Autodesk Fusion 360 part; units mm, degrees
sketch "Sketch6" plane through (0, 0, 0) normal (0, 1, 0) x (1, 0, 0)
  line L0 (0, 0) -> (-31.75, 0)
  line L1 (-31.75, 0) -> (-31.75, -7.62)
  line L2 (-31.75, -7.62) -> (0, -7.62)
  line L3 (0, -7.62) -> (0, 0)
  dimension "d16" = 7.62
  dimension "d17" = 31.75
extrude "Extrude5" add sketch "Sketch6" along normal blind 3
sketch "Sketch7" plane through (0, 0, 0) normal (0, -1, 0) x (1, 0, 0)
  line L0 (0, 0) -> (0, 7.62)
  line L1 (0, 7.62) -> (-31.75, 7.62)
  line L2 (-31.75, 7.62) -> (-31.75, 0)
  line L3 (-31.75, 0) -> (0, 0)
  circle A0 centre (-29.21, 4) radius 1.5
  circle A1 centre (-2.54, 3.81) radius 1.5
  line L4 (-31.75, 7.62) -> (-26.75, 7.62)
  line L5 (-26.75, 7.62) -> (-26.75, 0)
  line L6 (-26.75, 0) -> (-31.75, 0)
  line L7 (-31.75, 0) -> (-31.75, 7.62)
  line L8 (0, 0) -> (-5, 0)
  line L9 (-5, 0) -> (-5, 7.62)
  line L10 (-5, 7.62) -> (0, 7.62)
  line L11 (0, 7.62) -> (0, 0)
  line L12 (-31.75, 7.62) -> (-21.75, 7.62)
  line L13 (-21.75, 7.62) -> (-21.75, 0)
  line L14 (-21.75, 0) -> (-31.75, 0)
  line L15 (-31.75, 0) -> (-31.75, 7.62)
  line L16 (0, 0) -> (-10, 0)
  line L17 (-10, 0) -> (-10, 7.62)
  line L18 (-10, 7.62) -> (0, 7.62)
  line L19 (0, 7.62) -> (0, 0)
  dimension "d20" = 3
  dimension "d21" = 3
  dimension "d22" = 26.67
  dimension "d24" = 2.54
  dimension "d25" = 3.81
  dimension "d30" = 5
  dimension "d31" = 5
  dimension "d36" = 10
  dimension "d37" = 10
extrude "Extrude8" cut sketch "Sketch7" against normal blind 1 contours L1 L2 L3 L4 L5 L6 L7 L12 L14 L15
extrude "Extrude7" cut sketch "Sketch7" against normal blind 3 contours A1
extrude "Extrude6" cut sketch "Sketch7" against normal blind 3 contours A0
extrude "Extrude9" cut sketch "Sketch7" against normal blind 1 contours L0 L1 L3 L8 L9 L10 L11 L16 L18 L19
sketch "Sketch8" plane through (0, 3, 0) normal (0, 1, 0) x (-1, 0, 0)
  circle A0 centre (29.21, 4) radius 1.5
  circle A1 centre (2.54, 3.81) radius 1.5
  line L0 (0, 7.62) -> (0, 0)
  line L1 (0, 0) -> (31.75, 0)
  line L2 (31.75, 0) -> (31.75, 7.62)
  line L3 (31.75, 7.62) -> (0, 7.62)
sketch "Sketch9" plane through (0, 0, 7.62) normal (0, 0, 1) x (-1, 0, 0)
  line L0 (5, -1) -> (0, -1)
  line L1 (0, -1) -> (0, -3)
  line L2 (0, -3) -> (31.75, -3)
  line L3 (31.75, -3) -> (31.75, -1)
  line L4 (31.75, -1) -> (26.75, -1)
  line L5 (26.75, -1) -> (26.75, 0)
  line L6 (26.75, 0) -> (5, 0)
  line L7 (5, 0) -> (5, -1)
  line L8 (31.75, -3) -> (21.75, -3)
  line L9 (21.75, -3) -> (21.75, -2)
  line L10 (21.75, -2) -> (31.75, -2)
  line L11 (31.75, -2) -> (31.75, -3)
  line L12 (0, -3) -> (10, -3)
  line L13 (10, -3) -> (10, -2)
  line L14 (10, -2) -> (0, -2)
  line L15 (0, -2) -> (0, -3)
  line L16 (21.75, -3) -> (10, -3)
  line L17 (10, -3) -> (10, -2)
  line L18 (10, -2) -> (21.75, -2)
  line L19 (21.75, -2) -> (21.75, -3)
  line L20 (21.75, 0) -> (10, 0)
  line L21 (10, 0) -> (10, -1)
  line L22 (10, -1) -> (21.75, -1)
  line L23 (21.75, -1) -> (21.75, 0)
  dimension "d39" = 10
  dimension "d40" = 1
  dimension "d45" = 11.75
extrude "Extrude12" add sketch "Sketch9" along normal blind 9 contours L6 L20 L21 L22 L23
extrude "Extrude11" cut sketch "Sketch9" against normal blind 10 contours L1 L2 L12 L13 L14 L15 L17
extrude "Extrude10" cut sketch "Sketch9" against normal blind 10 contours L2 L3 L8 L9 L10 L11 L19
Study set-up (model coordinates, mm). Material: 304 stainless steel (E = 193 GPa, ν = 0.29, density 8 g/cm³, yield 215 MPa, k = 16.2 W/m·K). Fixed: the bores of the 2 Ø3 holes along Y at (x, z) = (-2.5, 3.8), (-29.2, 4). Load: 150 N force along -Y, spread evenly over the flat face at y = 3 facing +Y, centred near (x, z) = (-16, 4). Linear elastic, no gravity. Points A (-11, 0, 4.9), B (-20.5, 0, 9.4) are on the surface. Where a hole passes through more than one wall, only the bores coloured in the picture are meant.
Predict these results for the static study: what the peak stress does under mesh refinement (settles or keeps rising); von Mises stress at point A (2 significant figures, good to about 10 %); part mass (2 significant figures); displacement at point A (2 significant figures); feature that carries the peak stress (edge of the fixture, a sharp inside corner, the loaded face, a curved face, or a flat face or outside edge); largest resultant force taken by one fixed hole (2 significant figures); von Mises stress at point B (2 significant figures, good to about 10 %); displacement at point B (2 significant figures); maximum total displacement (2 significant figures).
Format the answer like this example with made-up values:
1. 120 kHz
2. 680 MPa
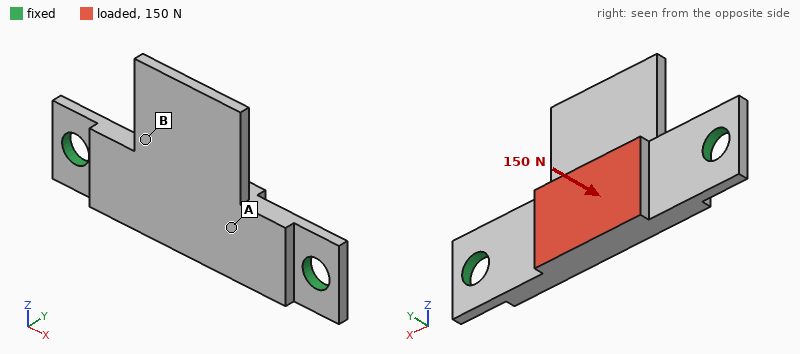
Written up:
1. keeps rising
2. 45 MPa
3. 4.7 g
4. 8.9 µm
5. edge of the fixture
6. 110 N
7. 18 MPa
8. 9.5 µm
9. 12 µm
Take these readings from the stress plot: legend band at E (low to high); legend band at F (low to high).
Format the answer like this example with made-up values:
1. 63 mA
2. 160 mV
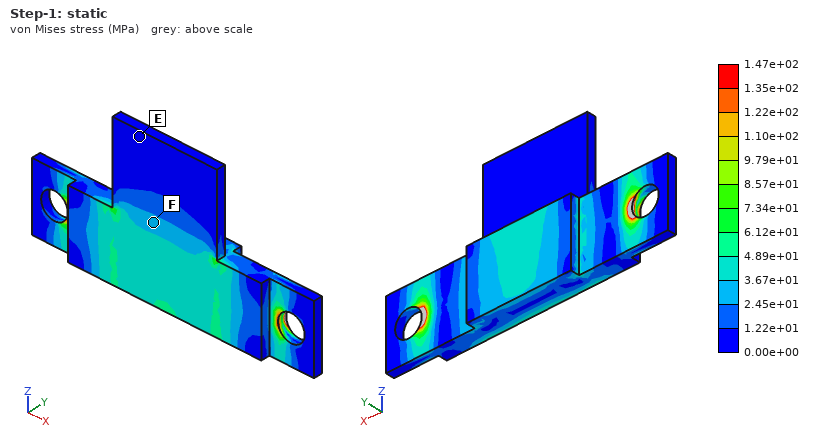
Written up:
1. 0.00e+00 to 1.22e+01 MPa
2. 2.45e+01 to 3.67e+01 MPa
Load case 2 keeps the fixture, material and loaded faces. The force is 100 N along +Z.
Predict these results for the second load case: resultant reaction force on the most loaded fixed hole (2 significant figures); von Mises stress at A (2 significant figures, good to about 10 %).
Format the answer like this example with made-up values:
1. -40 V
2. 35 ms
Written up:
1. 50 N
2. 8.5 MPa
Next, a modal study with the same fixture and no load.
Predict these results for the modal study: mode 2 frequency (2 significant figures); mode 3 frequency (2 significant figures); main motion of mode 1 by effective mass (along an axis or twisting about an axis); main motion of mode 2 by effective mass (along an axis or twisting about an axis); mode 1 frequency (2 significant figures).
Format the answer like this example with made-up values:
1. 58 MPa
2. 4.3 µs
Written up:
1. 12 kHz
2. 17 kHz
3. along Y
4. along Y
5. 6000 Hz
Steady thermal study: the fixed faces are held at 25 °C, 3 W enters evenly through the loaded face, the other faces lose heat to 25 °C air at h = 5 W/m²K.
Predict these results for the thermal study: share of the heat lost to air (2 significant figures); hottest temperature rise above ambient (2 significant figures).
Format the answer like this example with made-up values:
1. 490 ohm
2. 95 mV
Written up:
1. 5.4 %
2. 67 K
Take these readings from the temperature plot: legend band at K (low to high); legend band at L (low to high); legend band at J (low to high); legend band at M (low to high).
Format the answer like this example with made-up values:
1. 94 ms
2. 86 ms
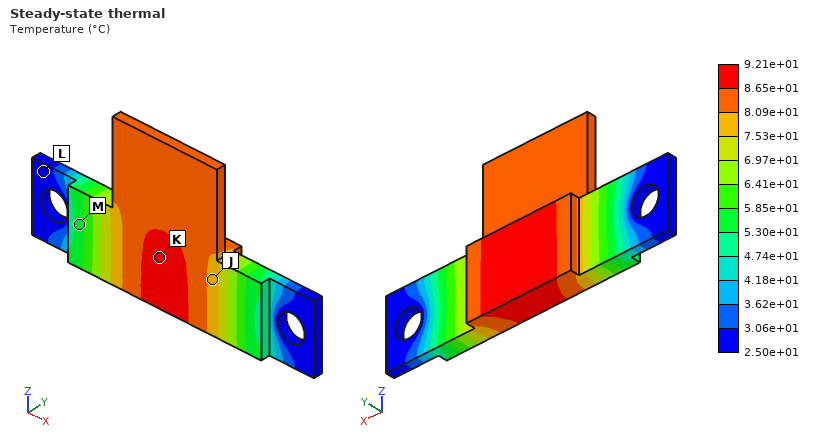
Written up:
1. 8.65e+01 to 9.21e+01 °C
2. 2.50e+01 to 3.06e+01 °C
3. 7.53e+01 to 8.09e+01 °C
4. 5.30e+01 to 5.85e+01 °C
